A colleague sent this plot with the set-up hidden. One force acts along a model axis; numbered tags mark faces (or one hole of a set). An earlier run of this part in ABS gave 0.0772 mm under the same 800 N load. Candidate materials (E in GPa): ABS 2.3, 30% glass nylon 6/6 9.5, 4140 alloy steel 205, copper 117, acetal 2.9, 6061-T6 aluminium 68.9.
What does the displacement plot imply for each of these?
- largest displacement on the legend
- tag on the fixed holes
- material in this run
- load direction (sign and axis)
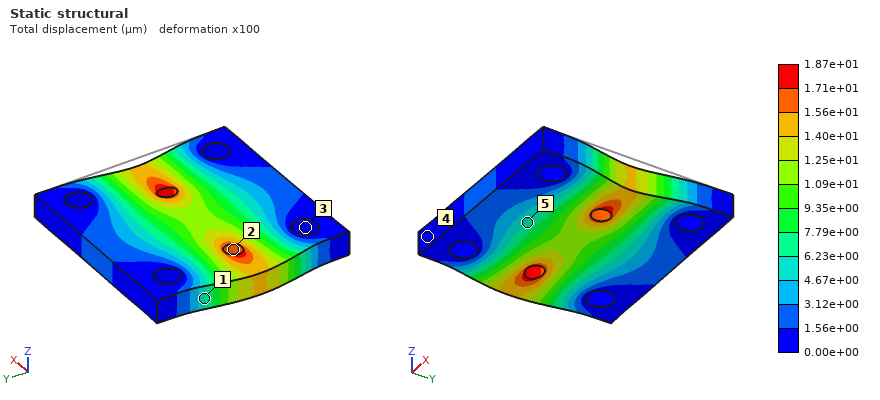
1.87e+01 µm
3
30% glass nylon 6/6
-X
